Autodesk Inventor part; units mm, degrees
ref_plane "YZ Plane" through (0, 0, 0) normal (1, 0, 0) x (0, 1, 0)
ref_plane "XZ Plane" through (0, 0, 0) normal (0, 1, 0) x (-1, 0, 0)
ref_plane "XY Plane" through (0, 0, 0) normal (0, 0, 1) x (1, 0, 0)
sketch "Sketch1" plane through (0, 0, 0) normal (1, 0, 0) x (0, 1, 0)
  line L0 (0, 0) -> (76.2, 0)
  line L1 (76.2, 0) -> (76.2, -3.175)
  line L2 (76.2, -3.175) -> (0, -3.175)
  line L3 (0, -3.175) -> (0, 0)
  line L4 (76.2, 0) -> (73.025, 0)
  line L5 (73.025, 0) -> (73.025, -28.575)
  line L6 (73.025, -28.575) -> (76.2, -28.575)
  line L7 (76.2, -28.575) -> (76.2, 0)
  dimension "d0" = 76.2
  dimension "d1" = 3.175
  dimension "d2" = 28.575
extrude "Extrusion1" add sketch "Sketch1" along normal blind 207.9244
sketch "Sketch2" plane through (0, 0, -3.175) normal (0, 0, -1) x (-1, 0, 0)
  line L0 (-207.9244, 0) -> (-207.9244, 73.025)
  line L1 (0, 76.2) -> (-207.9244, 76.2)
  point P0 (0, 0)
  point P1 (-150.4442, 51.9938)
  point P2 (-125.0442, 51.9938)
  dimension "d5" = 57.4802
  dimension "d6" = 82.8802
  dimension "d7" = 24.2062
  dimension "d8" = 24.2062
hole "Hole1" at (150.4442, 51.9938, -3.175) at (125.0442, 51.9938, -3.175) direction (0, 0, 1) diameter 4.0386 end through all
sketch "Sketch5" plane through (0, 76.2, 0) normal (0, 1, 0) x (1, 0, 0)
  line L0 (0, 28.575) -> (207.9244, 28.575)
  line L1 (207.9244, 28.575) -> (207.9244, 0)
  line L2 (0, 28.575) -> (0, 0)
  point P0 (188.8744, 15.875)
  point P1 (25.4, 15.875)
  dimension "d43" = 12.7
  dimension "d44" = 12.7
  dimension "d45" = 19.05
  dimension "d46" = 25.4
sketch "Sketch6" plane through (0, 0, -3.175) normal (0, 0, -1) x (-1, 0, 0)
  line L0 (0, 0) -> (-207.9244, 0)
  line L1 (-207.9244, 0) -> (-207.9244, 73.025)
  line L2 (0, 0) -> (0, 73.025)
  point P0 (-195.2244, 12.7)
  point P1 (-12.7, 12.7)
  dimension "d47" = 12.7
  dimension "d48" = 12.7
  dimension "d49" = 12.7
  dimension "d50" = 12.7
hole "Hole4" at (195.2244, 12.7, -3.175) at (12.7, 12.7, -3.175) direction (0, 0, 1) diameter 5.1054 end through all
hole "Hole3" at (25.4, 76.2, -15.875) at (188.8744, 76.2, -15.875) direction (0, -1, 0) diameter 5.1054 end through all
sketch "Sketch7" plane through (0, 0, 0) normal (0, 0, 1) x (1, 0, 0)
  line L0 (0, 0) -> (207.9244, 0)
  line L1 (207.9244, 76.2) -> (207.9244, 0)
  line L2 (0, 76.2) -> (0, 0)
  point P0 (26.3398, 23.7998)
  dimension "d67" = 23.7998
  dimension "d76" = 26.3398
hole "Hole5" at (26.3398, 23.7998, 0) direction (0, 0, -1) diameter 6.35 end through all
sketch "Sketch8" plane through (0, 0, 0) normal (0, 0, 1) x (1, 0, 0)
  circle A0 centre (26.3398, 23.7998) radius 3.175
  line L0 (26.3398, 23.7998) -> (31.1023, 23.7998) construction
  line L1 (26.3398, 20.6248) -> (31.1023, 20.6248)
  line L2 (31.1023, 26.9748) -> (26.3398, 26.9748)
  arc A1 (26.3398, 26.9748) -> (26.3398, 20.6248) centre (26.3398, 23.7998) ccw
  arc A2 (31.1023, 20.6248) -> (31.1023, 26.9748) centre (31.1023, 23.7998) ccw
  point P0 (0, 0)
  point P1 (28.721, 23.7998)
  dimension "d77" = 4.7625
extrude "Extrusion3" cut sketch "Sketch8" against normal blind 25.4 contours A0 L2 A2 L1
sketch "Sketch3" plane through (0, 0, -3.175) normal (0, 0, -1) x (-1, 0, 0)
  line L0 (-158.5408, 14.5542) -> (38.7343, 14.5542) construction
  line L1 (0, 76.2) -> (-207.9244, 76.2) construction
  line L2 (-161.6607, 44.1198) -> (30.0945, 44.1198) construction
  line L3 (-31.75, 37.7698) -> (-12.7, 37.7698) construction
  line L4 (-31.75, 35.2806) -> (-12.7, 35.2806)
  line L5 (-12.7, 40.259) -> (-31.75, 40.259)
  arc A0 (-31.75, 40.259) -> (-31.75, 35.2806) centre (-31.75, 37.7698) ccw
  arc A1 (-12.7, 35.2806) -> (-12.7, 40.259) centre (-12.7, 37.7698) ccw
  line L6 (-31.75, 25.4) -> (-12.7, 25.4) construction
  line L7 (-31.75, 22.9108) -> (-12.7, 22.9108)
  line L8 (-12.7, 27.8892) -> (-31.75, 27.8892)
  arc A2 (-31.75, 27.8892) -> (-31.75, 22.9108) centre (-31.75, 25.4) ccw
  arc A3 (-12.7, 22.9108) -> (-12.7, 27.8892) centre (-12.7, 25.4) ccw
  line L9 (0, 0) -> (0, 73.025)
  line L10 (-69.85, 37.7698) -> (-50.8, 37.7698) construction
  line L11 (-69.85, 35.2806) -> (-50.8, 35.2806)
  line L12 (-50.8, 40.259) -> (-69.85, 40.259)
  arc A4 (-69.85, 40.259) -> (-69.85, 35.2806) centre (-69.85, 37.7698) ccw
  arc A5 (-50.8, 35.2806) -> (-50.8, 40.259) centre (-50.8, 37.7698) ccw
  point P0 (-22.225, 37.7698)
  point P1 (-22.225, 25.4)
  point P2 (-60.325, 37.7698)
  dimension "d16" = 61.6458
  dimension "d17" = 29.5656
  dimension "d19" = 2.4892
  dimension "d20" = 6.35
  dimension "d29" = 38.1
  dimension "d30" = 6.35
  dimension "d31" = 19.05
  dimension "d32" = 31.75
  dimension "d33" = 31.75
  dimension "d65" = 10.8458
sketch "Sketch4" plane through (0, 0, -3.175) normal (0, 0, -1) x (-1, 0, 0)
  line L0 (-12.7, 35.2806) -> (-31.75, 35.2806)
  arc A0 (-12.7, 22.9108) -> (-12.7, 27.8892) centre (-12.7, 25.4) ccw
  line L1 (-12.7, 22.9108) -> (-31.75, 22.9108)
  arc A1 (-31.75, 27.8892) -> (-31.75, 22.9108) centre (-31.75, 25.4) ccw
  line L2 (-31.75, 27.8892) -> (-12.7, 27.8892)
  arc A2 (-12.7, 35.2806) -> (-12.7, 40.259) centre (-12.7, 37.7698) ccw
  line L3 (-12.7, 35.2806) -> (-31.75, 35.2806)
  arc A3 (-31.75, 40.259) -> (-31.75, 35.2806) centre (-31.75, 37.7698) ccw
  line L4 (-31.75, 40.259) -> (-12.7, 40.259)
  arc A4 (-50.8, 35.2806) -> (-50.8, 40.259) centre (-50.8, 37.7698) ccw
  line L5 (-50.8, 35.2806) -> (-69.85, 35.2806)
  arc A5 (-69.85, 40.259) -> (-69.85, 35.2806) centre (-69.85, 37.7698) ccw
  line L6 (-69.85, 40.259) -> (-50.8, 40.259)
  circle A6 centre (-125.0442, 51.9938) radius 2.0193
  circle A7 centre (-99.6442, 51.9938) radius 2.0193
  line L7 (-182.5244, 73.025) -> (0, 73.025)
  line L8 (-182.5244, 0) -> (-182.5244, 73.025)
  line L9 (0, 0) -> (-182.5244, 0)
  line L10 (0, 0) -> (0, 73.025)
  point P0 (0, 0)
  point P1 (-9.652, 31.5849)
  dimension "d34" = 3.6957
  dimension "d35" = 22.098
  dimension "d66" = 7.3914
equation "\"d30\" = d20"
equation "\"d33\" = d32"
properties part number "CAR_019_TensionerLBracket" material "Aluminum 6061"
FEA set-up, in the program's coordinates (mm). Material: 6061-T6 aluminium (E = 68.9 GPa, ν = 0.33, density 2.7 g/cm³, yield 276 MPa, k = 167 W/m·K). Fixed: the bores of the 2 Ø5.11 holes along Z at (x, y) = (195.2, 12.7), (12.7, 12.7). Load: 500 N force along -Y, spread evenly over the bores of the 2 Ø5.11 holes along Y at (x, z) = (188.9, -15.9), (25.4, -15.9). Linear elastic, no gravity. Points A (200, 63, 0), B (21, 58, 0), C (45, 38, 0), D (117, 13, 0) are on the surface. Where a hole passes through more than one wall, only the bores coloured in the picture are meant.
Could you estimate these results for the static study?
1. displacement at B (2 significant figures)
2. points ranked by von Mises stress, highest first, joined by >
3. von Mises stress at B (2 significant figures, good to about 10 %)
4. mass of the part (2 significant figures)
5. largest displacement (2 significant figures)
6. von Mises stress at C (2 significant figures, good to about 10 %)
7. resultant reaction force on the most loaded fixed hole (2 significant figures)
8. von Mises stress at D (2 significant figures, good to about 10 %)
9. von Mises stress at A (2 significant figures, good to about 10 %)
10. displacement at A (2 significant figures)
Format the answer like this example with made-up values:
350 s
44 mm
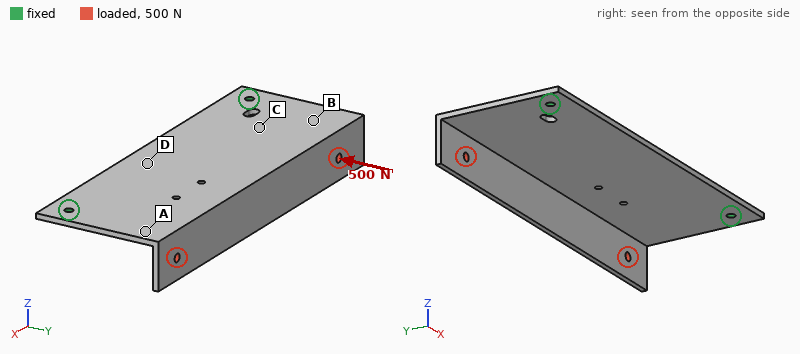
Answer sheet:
0.41 mm
A > B > C > D
25 MPa
180 g
0.96 mm
19 MPa
270 N
5.6 MPa
32 MPa
0.49 mm
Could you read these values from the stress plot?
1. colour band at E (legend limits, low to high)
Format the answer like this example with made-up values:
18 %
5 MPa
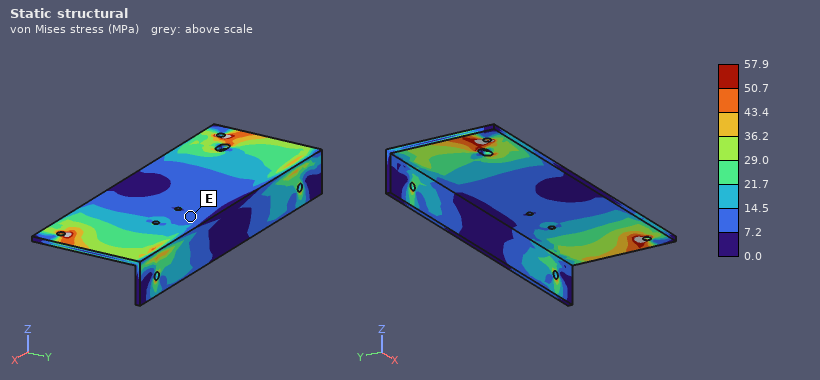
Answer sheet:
7.2 to 14.5 MPa
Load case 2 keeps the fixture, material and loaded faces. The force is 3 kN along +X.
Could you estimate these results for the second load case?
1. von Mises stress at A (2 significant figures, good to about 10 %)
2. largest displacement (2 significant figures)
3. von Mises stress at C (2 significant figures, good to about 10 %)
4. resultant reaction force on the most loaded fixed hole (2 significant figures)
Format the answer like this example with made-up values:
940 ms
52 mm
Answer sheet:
44 MPa
1.7 mm
37 MPa
1.8 kN
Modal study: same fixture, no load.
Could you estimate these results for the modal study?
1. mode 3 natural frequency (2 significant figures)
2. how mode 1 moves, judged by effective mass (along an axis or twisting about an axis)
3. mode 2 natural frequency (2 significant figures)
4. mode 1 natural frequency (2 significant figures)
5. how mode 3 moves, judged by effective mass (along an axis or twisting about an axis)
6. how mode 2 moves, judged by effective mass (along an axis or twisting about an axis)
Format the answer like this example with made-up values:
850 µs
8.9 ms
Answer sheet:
640 Hz
along Z
510 Hz
250 Hz
along Z
twisting about Y
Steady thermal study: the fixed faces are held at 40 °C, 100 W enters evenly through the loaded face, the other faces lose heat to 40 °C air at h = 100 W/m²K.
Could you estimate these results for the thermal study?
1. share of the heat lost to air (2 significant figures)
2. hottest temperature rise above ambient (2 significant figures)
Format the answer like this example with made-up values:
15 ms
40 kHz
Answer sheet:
82 %
80 K
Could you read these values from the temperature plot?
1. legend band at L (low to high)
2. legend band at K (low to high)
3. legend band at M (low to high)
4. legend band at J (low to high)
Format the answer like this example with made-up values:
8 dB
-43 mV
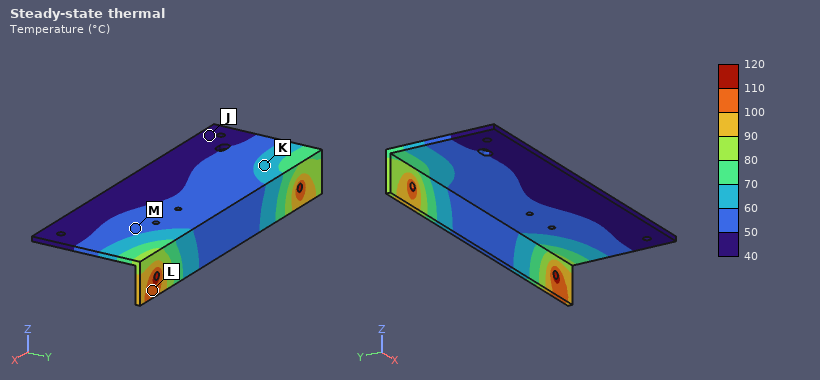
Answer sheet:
100 to 110 °C
60 to 70 °C
50 to 60 °C
40 to 50 °C
